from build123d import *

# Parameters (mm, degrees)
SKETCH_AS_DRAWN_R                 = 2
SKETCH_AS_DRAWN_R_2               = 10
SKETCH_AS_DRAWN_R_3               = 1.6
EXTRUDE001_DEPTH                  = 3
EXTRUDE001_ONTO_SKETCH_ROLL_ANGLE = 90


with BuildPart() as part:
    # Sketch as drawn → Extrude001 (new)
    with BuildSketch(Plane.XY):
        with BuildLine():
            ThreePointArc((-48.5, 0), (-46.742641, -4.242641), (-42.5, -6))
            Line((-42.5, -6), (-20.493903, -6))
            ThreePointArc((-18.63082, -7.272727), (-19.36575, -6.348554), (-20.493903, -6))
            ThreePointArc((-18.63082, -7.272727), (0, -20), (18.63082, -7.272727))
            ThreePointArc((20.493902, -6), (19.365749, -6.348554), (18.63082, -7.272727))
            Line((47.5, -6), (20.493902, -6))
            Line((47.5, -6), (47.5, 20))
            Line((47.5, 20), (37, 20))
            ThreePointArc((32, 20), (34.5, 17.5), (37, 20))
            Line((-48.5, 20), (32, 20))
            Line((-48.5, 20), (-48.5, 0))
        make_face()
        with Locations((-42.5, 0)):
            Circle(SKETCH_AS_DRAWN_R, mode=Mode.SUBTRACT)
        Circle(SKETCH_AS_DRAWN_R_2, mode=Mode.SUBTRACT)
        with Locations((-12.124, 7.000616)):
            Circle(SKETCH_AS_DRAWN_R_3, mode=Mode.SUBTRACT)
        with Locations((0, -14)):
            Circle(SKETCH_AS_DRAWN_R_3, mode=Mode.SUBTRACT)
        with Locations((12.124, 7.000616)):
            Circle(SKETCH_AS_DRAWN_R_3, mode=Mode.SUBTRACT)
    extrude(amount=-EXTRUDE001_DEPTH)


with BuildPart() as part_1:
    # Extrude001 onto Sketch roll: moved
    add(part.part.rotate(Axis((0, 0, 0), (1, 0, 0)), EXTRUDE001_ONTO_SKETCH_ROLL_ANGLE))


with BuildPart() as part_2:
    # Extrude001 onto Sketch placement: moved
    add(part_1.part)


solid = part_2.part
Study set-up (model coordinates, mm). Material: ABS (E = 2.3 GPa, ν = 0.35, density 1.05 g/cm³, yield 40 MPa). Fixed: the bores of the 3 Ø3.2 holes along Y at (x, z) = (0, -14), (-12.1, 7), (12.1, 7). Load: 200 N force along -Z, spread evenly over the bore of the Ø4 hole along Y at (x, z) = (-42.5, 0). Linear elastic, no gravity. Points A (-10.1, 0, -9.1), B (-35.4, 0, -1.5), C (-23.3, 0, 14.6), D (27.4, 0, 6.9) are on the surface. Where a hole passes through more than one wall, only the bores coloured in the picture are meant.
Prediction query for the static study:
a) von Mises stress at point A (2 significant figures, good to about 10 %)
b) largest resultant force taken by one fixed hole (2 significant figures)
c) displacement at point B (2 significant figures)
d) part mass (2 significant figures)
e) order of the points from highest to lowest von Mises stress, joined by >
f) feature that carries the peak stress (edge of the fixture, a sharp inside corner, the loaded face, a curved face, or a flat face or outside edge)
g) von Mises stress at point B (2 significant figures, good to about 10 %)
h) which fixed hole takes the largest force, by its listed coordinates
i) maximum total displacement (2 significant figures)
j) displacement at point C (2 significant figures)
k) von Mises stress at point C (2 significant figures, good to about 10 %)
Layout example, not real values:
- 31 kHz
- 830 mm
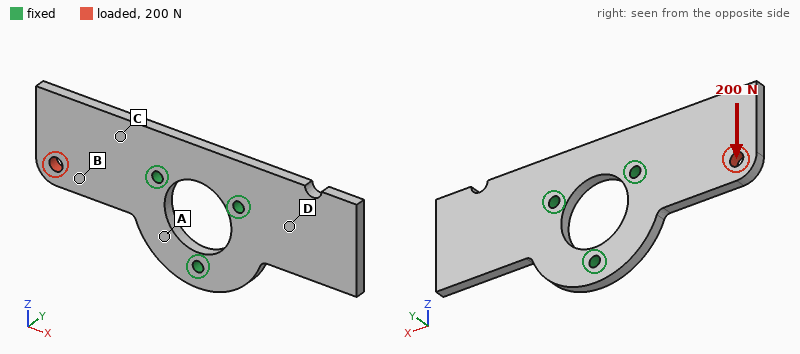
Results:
- 11 MPa
- 250 N
- 0.34 mm
- 7.9 g
- A > C > B > D
- a curved face
- 5.1 MPa
- (0, -14)
- 0.57 mm
- 0.16 mm
- 6.8 MPa
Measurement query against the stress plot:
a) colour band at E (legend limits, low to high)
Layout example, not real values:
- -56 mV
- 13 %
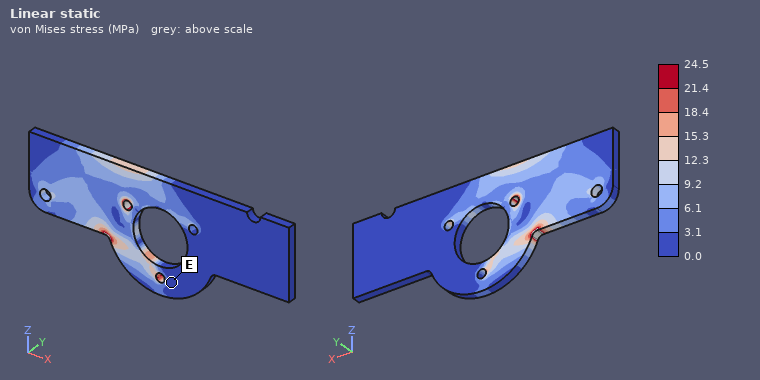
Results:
- 0.0 to 3.1 MPa
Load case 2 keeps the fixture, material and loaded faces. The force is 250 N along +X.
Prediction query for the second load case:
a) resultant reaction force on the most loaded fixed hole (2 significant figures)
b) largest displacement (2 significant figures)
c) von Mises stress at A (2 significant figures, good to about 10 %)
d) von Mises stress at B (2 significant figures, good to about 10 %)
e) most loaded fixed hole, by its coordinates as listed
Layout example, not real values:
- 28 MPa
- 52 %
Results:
- 170 N
- 0.19 mm
- 4.9 MPa
- 7.0 MPa
- (-12.1, 7)
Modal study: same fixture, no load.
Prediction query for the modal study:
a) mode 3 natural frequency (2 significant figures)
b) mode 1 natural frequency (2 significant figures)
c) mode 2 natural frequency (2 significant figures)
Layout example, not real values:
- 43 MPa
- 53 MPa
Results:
- 1400 Hz
- 540 Hz
- 560 Hz
